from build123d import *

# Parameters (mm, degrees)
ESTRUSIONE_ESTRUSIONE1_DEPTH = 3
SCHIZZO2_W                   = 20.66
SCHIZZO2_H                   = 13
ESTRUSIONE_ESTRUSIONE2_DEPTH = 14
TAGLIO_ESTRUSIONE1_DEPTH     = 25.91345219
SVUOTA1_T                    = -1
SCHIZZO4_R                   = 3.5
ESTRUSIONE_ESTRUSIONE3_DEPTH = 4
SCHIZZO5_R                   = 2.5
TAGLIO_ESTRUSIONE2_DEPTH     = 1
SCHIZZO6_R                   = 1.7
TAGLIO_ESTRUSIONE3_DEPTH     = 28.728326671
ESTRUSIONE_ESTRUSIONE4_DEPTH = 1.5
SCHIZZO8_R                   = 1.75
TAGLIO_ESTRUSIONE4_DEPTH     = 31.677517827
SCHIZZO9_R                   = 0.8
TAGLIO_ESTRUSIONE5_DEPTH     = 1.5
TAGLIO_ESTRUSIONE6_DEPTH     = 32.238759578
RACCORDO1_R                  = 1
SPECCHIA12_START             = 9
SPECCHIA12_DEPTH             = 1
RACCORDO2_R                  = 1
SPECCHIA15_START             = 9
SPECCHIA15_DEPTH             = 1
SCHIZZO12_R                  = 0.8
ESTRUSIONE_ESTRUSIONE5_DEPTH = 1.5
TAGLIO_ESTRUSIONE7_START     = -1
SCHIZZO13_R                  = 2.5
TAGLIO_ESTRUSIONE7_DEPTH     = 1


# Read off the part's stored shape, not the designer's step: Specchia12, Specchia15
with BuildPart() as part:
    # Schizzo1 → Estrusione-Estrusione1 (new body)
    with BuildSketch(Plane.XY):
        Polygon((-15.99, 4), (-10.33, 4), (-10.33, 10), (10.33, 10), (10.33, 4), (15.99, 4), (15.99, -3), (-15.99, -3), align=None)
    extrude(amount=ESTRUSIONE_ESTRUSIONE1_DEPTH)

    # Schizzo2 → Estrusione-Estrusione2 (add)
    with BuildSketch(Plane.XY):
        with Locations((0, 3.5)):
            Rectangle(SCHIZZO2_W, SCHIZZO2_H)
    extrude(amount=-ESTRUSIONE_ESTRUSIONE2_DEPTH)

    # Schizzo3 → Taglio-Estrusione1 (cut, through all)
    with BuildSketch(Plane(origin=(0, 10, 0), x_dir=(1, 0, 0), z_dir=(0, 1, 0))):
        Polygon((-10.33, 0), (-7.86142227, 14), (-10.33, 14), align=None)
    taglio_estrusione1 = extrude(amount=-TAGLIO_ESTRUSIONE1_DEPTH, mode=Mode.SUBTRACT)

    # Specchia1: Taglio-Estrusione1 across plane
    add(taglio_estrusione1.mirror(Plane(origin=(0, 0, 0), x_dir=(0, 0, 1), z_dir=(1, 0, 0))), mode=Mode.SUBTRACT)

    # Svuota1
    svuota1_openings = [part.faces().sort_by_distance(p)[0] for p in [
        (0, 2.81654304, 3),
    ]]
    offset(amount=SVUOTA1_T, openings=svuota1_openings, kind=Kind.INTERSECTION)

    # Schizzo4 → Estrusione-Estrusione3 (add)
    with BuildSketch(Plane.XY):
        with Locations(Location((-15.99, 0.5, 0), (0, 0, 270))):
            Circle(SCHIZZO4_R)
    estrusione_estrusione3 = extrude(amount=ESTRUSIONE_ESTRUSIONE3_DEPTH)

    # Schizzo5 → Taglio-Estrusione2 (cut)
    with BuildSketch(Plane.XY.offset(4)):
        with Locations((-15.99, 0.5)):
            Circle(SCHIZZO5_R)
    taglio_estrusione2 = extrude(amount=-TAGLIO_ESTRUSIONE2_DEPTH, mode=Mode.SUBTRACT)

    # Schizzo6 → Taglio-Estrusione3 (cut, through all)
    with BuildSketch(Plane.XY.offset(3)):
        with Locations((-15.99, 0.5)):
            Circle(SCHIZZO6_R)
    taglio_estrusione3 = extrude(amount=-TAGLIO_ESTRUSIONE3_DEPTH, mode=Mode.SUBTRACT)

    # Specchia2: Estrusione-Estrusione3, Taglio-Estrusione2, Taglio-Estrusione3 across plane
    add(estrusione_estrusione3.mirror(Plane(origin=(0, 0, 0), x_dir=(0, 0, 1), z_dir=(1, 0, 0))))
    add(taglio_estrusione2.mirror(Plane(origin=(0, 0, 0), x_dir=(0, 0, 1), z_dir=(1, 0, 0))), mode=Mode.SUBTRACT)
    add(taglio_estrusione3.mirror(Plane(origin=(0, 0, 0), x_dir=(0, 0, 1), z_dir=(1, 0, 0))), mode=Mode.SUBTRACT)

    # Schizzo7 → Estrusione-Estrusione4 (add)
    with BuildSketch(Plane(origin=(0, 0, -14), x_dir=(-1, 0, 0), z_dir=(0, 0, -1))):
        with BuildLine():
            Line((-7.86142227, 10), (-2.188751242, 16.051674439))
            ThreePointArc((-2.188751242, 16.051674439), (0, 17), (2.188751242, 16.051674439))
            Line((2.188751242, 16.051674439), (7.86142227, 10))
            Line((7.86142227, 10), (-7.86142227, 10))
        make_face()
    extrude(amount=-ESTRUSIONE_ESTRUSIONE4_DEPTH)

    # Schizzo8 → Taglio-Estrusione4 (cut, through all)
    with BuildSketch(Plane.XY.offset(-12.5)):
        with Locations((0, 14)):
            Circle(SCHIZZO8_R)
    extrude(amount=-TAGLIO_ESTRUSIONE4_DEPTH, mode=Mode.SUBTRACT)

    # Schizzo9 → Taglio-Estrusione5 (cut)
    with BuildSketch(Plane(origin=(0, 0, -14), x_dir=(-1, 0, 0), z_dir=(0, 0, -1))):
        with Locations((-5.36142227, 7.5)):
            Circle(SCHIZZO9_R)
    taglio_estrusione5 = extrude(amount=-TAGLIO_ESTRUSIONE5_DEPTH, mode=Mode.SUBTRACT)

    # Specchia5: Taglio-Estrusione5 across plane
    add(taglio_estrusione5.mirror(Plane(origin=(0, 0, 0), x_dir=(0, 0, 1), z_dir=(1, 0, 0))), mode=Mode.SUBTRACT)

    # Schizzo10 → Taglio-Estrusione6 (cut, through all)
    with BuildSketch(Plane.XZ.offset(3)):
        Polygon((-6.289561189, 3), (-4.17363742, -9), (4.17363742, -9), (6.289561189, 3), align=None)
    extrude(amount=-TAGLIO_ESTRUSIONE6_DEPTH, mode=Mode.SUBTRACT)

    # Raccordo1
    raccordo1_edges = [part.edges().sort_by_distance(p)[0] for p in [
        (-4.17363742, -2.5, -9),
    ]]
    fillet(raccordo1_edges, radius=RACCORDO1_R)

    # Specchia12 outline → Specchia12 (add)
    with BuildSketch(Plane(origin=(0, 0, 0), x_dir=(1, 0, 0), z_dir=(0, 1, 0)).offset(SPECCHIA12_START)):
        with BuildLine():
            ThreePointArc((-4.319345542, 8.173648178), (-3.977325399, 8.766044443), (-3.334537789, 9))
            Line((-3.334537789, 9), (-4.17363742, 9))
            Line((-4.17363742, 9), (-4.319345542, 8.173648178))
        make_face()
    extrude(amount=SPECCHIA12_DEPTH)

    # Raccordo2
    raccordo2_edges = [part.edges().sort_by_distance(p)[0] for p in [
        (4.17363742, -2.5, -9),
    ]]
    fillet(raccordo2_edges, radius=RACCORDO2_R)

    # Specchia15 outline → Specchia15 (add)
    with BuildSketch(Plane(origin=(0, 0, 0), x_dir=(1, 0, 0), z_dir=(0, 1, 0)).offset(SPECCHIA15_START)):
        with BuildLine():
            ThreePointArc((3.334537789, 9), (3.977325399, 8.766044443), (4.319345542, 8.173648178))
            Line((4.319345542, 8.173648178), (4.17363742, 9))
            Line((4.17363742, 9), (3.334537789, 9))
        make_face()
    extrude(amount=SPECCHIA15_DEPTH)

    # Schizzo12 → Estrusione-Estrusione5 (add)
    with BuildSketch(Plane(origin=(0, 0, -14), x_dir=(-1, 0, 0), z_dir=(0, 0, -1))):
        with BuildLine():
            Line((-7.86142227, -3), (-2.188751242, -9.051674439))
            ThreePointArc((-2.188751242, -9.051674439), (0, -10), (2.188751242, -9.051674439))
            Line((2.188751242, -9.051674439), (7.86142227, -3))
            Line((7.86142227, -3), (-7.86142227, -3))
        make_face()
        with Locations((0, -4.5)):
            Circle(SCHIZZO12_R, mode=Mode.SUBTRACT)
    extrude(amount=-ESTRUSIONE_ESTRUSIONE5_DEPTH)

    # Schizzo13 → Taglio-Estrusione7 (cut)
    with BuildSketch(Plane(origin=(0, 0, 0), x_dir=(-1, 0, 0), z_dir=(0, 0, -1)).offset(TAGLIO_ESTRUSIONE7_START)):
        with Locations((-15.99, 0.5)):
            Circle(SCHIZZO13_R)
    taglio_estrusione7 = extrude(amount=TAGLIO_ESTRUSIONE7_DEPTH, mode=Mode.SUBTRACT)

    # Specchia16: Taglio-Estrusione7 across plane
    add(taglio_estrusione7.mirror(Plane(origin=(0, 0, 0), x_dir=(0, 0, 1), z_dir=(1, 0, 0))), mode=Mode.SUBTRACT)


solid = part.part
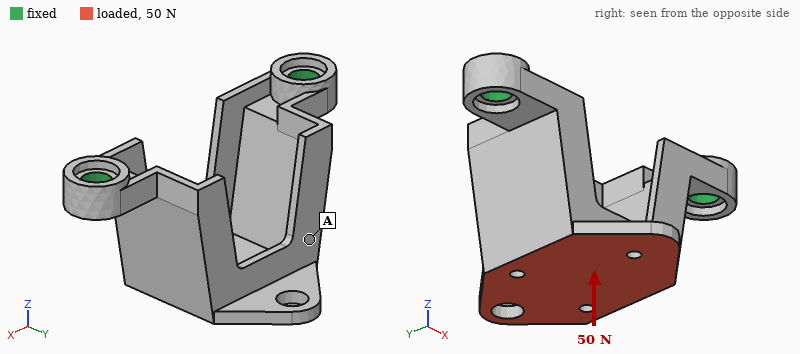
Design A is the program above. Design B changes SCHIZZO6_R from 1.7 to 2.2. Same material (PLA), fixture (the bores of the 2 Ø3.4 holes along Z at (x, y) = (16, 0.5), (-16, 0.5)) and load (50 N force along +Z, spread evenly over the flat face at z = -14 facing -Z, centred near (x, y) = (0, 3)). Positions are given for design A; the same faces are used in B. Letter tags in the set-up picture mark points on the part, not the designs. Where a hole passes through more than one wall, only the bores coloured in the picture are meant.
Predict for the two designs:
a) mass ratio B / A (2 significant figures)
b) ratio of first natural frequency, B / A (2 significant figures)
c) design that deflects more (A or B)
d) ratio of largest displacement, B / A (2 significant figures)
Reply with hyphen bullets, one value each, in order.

- 0.98
- 1.1
- A
- 0.89
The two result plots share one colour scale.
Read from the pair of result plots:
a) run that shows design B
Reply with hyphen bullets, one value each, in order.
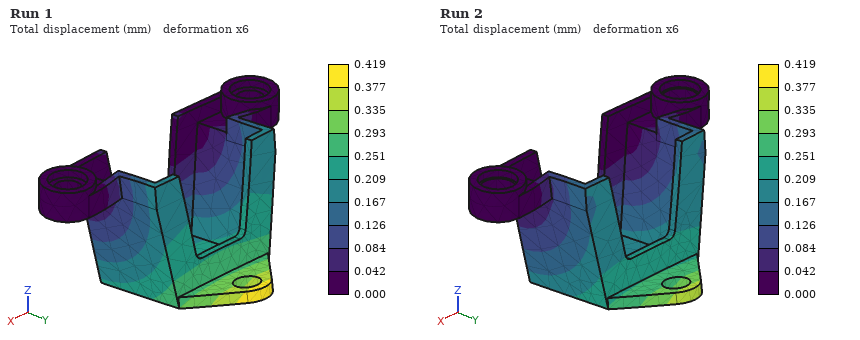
- Run 2
